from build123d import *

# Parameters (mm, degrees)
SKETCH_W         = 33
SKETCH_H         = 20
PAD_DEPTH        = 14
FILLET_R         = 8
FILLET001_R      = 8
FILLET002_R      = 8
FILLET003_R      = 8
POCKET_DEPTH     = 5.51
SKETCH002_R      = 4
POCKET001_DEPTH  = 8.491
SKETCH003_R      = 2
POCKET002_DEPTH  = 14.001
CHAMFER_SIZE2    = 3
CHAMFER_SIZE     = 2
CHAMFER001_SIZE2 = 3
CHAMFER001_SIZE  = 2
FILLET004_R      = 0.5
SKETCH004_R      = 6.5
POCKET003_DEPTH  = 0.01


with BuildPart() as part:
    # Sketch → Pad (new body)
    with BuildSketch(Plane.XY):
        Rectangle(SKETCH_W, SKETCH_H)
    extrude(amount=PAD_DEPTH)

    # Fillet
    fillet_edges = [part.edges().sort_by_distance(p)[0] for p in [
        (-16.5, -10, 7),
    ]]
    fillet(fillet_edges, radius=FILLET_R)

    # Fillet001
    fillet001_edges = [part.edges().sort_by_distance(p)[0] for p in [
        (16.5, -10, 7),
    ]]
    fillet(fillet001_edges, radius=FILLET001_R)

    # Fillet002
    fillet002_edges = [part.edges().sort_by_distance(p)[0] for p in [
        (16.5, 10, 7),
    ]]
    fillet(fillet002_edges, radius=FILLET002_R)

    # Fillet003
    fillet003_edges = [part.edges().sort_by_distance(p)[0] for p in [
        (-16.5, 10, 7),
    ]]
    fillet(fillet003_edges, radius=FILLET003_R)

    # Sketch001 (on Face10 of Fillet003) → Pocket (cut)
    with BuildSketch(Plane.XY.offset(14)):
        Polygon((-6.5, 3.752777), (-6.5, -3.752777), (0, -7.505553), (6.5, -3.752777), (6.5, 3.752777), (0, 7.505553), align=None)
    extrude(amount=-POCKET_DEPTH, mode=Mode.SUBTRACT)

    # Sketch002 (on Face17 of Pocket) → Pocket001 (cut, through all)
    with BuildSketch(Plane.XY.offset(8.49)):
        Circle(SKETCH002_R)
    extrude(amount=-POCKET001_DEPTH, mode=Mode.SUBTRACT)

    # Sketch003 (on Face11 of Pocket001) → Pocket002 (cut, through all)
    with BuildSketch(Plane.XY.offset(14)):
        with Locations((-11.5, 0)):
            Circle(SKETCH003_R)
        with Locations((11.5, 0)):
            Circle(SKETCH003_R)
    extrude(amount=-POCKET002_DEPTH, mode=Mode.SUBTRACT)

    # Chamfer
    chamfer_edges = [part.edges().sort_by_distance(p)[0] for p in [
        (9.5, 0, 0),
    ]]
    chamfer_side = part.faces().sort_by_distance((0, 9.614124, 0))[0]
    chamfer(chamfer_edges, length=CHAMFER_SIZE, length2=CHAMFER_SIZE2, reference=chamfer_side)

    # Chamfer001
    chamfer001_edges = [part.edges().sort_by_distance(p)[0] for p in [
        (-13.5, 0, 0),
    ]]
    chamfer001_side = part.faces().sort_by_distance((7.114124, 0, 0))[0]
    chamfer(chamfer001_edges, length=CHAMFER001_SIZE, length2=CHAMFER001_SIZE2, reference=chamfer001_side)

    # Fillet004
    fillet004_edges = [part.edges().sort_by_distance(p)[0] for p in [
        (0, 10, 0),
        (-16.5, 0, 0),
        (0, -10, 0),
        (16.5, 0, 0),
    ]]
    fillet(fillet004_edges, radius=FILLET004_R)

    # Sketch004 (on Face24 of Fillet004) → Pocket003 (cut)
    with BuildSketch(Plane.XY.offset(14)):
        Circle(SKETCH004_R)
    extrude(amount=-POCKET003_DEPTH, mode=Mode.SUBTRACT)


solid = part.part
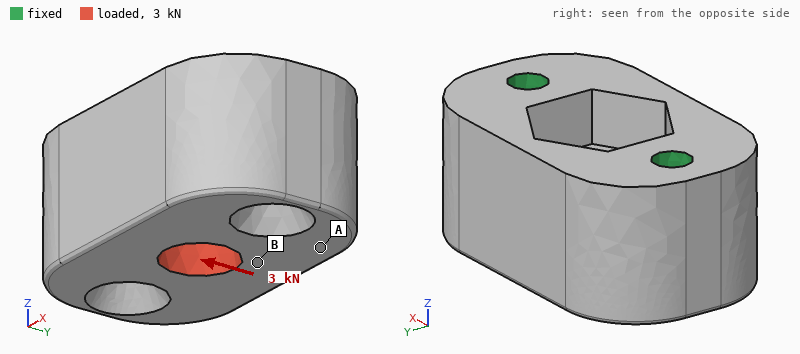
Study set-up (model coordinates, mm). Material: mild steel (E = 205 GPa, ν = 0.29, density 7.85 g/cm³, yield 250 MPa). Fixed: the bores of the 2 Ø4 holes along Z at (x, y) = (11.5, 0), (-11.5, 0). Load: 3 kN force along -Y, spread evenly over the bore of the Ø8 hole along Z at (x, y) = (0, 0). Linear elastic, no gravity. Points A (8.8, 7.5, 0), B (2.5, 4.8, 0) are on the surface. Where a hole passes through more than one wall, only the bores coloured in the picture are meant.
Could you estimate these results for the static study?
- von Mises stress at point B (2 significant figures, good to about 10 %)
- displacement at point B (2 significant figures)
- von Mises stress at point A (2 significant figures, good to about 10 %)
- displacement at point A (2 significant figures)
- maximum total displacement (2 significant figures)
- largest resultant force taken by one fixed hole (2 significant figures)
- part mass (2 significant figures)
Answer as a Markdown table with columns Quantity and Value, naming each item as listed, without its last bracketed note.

| Quantity | Value |
|---|---|
| von Mises stress at point B | 17 MPa |
| displacement at point B | 1.8 µm |
| von Mises stress at point A | 8.1 MPa |
| displacement at point A | 1.0 µm |
| maximum total displacement | 2.1 µm |
| largest resultant force taken by one fixed hole | 1.5 kN |
| part mass | 53 g |
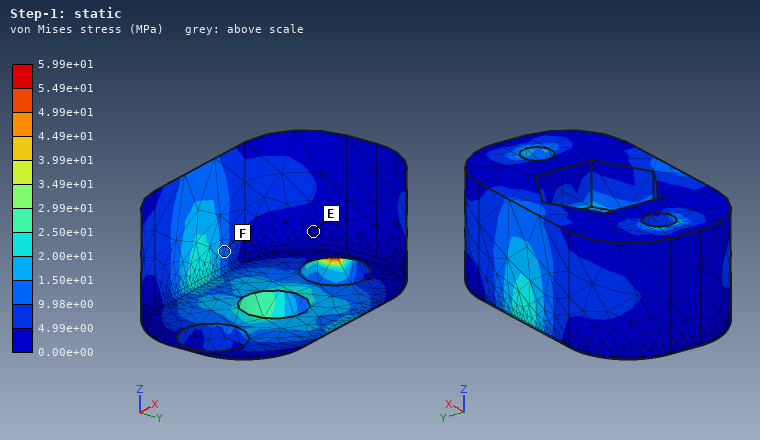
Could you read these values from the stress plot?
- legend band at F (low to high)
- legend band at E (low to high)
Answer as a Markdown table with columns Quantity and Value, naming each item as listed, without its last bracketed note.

| Quantity | Value |
|---|---|
| legend band at F | 9.98e+00 to 1.50e+01 MPa |
| legend band at E | 0.00e+00 to 4.99e+00 MPa |
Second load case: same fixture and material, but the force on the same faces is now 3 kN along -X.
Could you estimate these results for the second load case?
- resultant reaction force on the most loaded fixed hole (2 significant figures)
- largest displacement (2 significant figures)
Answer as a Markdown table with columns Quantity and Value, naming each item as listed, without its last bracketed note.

| Quantity | Value |
|---|---|
| resultant reaction force on the most loaded fixed hole | 1.5 kN |
| largest displacement | 0.90 µm |
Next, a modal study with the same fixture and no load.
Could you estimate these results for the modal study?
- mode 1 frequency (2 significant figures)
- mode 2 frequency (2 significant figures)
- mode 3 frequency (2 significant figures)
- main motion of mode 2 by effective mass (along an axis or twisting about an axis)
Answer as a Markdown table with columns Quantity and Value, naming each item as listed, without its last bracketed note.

| Quantity | Value |
|---|---|
| mode 1 frequency | 40 kHz |
| mode 2 frequency | 46 kHz |
| mode 3 frequency | 54 kHz |
| main motion of mode 2 by effective mass | along Z |
